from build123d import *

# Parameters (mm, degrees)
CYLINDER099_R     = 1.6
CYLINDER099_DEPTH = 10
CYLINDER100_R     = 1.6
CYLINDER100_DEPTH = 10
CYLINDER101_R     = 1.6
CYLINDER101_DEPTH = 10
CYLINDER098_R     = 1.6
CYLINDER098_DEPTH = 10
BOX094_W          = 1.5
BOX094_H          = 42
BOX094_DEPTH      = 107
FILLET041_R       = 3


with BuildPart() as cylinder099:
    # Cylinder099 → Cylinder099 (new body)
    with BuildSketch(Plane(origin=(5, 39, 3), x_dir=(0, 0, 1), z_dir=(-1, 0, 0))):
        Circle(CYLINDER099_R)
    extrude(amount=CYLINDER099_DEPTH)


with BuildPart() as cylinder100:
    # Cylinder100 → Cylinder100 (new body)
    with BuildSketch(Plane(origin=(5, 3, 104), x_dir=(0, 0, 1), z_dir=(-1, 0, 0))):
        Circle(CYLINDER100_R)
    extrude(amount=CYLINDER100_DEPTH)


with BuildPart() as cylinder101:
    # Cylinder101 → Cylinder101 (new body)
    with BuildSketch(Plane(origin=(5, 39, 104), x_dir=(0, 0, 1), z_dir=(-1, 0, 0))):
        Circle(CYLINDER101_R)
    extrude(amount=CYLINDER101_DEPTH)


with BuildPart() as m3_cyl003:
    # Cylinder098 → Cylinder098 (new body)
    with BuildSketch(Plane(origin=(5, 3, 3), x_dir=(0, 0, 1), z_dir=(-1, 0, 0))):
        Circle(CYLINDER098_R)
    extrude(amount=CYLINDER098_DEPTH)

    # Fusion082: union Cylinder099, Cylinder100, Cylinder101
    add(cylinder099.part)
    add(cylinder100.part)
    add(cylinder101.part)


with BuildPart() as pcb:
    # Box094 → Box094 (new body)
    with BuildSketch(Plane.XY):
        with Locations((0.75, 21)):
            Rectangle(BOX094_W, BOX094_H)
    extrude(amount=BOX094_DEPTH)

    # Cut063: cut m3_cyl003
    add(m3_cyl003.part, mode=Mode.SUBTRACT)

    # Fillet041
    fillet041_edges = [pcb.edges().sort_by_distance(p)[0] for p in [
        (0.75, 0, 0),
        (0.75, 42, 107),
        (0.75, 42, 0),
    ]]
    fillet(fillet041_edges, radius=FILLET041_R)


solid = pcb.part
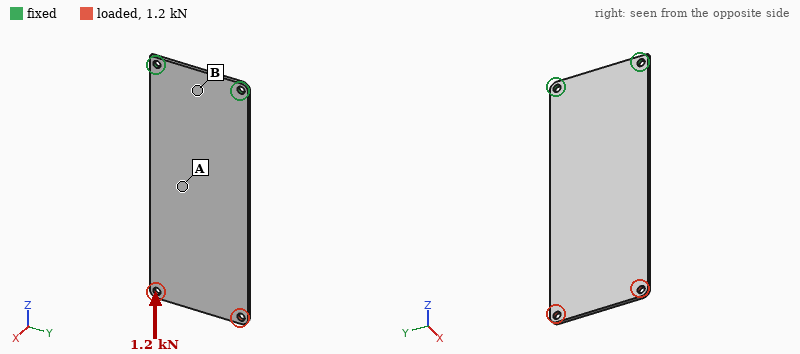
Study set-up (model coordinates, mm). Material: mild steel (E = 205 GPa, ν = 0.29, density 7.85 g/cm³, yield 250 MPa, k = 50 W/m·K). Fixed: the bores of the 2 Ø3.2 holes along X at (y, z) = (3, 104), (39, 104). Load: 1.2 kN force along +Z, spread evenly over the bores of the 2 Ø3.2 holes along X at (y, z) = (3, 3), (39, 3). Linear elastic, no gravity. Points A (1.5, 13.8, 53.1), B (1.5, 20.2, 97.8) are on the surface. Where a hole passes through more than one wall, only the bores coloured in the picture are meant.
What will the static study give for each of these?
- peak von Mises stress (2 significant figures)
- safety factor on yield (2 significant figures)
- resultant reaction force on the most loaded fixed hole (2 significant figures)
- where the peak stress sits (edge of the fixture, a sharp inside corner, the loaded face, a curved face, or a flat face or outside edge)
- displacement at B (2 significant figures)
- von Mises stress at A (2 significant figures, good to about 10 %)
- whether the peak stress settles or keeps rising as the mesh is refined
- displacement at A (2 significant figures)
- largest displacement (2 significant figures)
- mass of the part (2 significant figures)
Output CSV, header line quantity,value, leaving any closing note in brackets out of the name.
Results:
quantity,value
peak von Mises stress,190 MPa
safety factor on yield,1.3
resultant reaction force on the most loaded fixed hole,630 N
where the peak stress sits,the loaded face
displacement at B,3.1 µm
von Mises stress at A,19 MPa
whether the peak stress settles or keeps rising as the mesh is refined,settles
displacement at A,6.3 µm
largest displacement,15 µm
mass of the part,52 g
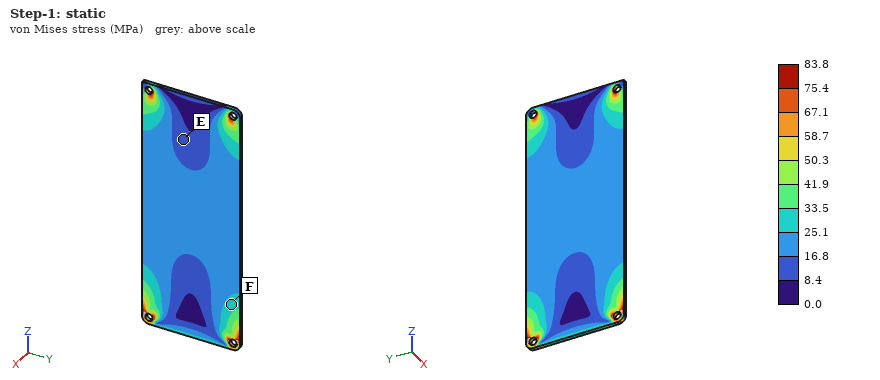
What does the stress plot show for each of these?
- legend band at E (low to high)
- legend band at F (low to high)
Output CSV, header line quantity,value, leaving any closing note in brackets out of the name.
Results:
quantity,value
legend band at E,8.4 to 16.8 MPa
legend band at F,25.1 to 33.5 MPa
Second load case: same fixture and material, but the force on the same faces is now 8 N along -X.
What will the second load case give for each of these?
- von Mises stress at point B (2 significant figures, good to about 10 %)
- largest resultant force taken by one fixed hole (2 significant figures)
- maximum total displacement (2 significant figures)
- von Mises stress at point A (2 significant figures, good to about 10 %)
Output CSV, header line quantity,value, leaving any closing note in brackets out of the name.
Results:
quantity,value
von Mises stress at point B,30 MPa
largest resultant force taken by one fixed hole,4.0 N
maximum total displacement,1.3 mm
von Mises stress at point A,25 MPa
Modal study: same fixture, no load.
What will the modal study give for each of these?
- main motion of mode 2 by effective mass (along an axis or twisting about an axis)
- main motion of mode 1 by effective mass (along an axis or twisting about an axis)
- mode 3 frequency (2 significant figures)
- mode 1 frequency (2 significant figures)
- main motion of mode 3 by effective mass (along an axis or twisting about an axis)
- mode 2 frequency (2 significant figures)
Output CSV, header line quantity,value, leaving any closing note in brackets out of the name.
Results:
quantity,value
main motion of mode 2 by effective mass,twisting about Z
main motion of mode 1 by effective mass,along X
mode 3 frequency,690 Hz
mode 1 frequency,110 Hz
main motion of mode 3 by effective mass,along X
mode 2 frequency,610 Hz
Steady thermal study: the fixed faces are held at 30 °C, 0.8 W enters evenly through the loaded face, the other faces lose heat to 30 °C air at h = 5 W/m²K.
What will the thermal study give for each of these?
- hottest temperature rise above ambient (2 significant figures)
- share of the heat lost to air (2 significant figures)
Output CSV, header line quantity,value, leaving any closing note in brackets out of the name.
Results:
quantity,value
hottest temperature rise above ambient,21 K
share of the heat lost to air,49 %
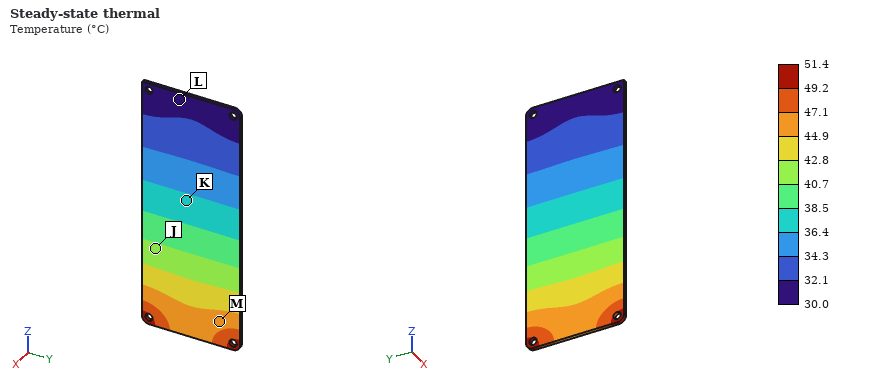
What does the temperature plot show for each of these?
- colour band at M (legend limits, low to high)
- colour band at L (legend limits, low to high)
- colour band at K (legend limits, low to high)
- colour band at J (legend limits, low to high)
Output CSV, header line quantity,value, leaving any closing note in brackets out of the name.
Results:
quantity,value
colour band at M,44.9 to 47.1 °C
colour band at L,30.0 to 32.1 °C
colour band at K,36.4 to 38.5 °C
colour band at J,40.7 to 42.8 °C
